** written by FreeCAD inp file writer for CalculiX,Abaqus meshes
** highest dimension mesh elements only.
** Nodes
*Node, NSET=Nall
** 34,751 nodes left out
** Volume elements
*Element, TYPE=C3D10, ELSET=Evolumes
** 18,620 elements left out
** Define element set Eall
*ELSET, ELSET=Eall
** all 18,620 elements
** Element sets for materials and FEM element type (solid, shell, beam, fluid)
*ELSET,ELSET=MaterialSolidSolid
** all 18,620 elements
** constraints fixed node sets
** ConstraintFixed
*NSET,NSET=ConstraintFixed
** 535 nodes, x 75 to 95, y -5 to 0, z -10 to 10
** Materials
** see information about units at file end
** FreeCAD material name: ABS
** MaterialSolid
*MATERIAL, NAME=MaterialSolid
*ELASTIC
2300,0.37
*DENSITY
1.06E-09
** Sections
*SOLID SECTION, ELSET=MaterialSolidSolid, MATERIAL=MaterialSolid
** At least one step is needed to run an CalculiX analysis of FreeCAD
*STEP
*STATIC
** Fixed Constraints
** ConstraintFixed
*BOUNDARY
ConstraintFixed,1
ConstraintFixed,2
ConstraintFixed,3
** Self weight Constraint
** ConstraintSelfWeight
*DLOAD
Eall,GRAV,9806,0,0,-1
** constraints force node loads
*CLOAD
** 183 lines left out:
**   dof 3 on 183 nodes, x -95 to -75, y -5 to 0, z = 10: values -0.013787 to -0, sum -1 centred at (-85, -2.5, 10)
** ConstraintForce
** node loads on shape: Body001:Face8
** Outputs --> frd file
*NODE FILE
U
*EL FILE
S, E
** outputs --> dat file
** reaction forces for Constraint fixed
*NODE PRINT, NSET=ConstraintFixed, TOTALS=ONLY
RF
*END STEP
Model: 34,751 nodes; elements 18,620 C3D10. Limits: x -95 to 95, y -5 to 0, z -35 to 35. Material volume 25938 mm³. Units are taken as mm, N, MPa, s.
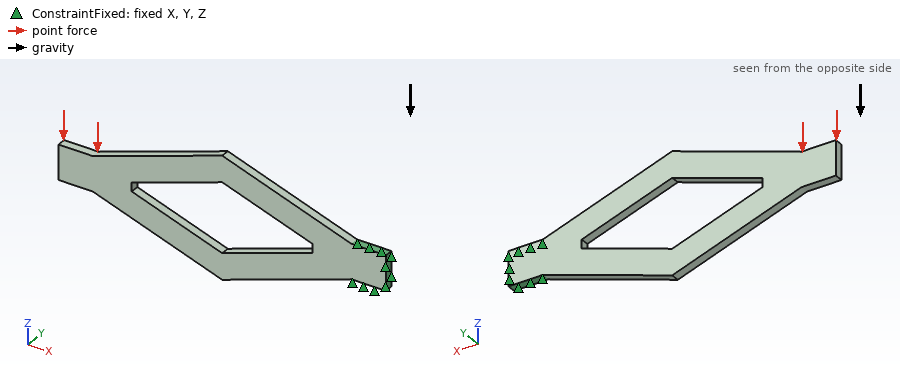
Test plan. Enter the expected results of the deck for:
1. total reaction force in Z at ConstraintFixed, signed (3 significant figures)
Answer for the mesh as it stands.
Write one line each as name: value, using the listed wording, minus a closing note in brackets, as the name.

total reaction force in Z at ConstraintFixed, signed: 1.27 N
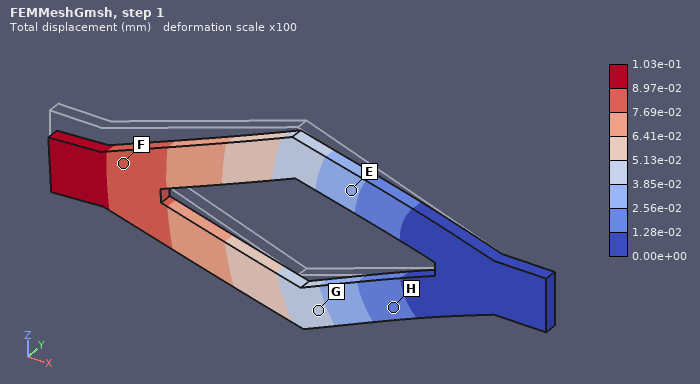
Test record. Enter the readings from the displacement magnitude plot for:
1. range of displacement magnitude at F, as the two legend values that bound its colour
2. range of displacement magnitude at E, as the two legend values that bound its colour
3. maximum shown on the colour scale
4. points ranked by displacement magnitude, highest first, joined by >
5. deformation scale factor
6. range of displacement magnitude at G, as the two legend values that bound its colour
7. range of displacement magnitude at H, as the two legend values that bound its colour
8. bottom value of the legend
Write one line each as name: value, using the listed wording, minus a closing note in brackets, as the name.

range of displacement magnitude at F, as the two legend values that bound its colour: 7.69e-02 to 8.97e-02 mm
range of displacement magnitude at E, as the two legend values that bound its colour: 2.56e-02 to 3.85e-02 mm
maximum shown on the colour scale: 1.03e-01 mm
points ranked by displacement magnitude, highest first, joined by >: F > G > E > H
deformation scale factor: 100
range of displacement magnitude at G, as the two legend values that bound its colour: 3.85e-02 to 5.13e-02 mm
range of displacement magnitude at H, as the two legend values that bound its colour: 1.28e-02 to 2.56e-02 mm
bottom value of the legend: 0.00e+00 mm
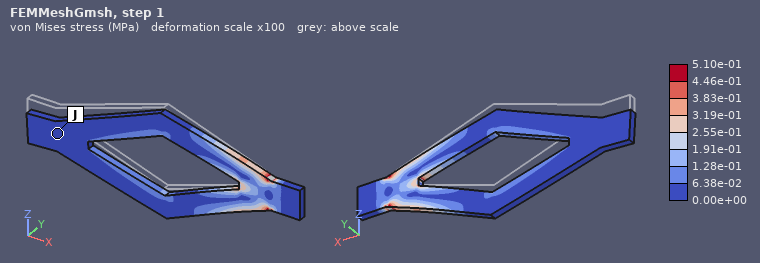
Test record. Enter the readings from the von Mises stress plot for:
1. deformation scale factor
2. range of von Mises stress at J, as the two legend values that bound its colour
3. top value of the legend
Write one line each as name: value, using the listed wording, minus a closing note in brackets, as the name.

deformation scale factor: 100
range of von Mises stress at J, as the two legend values that bound its colour: 0.00e+00 to 6.38e-02 MPa
top value of the legend: 5.10e-01 MPa
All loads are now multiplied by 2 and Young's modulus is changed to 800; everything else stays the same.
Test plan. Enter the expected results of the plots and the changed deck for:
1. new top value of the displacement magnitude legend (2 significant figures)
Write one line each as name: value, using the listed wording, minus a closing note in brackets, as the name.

new top value of the displacement magnitude legend: 0.59 mm
